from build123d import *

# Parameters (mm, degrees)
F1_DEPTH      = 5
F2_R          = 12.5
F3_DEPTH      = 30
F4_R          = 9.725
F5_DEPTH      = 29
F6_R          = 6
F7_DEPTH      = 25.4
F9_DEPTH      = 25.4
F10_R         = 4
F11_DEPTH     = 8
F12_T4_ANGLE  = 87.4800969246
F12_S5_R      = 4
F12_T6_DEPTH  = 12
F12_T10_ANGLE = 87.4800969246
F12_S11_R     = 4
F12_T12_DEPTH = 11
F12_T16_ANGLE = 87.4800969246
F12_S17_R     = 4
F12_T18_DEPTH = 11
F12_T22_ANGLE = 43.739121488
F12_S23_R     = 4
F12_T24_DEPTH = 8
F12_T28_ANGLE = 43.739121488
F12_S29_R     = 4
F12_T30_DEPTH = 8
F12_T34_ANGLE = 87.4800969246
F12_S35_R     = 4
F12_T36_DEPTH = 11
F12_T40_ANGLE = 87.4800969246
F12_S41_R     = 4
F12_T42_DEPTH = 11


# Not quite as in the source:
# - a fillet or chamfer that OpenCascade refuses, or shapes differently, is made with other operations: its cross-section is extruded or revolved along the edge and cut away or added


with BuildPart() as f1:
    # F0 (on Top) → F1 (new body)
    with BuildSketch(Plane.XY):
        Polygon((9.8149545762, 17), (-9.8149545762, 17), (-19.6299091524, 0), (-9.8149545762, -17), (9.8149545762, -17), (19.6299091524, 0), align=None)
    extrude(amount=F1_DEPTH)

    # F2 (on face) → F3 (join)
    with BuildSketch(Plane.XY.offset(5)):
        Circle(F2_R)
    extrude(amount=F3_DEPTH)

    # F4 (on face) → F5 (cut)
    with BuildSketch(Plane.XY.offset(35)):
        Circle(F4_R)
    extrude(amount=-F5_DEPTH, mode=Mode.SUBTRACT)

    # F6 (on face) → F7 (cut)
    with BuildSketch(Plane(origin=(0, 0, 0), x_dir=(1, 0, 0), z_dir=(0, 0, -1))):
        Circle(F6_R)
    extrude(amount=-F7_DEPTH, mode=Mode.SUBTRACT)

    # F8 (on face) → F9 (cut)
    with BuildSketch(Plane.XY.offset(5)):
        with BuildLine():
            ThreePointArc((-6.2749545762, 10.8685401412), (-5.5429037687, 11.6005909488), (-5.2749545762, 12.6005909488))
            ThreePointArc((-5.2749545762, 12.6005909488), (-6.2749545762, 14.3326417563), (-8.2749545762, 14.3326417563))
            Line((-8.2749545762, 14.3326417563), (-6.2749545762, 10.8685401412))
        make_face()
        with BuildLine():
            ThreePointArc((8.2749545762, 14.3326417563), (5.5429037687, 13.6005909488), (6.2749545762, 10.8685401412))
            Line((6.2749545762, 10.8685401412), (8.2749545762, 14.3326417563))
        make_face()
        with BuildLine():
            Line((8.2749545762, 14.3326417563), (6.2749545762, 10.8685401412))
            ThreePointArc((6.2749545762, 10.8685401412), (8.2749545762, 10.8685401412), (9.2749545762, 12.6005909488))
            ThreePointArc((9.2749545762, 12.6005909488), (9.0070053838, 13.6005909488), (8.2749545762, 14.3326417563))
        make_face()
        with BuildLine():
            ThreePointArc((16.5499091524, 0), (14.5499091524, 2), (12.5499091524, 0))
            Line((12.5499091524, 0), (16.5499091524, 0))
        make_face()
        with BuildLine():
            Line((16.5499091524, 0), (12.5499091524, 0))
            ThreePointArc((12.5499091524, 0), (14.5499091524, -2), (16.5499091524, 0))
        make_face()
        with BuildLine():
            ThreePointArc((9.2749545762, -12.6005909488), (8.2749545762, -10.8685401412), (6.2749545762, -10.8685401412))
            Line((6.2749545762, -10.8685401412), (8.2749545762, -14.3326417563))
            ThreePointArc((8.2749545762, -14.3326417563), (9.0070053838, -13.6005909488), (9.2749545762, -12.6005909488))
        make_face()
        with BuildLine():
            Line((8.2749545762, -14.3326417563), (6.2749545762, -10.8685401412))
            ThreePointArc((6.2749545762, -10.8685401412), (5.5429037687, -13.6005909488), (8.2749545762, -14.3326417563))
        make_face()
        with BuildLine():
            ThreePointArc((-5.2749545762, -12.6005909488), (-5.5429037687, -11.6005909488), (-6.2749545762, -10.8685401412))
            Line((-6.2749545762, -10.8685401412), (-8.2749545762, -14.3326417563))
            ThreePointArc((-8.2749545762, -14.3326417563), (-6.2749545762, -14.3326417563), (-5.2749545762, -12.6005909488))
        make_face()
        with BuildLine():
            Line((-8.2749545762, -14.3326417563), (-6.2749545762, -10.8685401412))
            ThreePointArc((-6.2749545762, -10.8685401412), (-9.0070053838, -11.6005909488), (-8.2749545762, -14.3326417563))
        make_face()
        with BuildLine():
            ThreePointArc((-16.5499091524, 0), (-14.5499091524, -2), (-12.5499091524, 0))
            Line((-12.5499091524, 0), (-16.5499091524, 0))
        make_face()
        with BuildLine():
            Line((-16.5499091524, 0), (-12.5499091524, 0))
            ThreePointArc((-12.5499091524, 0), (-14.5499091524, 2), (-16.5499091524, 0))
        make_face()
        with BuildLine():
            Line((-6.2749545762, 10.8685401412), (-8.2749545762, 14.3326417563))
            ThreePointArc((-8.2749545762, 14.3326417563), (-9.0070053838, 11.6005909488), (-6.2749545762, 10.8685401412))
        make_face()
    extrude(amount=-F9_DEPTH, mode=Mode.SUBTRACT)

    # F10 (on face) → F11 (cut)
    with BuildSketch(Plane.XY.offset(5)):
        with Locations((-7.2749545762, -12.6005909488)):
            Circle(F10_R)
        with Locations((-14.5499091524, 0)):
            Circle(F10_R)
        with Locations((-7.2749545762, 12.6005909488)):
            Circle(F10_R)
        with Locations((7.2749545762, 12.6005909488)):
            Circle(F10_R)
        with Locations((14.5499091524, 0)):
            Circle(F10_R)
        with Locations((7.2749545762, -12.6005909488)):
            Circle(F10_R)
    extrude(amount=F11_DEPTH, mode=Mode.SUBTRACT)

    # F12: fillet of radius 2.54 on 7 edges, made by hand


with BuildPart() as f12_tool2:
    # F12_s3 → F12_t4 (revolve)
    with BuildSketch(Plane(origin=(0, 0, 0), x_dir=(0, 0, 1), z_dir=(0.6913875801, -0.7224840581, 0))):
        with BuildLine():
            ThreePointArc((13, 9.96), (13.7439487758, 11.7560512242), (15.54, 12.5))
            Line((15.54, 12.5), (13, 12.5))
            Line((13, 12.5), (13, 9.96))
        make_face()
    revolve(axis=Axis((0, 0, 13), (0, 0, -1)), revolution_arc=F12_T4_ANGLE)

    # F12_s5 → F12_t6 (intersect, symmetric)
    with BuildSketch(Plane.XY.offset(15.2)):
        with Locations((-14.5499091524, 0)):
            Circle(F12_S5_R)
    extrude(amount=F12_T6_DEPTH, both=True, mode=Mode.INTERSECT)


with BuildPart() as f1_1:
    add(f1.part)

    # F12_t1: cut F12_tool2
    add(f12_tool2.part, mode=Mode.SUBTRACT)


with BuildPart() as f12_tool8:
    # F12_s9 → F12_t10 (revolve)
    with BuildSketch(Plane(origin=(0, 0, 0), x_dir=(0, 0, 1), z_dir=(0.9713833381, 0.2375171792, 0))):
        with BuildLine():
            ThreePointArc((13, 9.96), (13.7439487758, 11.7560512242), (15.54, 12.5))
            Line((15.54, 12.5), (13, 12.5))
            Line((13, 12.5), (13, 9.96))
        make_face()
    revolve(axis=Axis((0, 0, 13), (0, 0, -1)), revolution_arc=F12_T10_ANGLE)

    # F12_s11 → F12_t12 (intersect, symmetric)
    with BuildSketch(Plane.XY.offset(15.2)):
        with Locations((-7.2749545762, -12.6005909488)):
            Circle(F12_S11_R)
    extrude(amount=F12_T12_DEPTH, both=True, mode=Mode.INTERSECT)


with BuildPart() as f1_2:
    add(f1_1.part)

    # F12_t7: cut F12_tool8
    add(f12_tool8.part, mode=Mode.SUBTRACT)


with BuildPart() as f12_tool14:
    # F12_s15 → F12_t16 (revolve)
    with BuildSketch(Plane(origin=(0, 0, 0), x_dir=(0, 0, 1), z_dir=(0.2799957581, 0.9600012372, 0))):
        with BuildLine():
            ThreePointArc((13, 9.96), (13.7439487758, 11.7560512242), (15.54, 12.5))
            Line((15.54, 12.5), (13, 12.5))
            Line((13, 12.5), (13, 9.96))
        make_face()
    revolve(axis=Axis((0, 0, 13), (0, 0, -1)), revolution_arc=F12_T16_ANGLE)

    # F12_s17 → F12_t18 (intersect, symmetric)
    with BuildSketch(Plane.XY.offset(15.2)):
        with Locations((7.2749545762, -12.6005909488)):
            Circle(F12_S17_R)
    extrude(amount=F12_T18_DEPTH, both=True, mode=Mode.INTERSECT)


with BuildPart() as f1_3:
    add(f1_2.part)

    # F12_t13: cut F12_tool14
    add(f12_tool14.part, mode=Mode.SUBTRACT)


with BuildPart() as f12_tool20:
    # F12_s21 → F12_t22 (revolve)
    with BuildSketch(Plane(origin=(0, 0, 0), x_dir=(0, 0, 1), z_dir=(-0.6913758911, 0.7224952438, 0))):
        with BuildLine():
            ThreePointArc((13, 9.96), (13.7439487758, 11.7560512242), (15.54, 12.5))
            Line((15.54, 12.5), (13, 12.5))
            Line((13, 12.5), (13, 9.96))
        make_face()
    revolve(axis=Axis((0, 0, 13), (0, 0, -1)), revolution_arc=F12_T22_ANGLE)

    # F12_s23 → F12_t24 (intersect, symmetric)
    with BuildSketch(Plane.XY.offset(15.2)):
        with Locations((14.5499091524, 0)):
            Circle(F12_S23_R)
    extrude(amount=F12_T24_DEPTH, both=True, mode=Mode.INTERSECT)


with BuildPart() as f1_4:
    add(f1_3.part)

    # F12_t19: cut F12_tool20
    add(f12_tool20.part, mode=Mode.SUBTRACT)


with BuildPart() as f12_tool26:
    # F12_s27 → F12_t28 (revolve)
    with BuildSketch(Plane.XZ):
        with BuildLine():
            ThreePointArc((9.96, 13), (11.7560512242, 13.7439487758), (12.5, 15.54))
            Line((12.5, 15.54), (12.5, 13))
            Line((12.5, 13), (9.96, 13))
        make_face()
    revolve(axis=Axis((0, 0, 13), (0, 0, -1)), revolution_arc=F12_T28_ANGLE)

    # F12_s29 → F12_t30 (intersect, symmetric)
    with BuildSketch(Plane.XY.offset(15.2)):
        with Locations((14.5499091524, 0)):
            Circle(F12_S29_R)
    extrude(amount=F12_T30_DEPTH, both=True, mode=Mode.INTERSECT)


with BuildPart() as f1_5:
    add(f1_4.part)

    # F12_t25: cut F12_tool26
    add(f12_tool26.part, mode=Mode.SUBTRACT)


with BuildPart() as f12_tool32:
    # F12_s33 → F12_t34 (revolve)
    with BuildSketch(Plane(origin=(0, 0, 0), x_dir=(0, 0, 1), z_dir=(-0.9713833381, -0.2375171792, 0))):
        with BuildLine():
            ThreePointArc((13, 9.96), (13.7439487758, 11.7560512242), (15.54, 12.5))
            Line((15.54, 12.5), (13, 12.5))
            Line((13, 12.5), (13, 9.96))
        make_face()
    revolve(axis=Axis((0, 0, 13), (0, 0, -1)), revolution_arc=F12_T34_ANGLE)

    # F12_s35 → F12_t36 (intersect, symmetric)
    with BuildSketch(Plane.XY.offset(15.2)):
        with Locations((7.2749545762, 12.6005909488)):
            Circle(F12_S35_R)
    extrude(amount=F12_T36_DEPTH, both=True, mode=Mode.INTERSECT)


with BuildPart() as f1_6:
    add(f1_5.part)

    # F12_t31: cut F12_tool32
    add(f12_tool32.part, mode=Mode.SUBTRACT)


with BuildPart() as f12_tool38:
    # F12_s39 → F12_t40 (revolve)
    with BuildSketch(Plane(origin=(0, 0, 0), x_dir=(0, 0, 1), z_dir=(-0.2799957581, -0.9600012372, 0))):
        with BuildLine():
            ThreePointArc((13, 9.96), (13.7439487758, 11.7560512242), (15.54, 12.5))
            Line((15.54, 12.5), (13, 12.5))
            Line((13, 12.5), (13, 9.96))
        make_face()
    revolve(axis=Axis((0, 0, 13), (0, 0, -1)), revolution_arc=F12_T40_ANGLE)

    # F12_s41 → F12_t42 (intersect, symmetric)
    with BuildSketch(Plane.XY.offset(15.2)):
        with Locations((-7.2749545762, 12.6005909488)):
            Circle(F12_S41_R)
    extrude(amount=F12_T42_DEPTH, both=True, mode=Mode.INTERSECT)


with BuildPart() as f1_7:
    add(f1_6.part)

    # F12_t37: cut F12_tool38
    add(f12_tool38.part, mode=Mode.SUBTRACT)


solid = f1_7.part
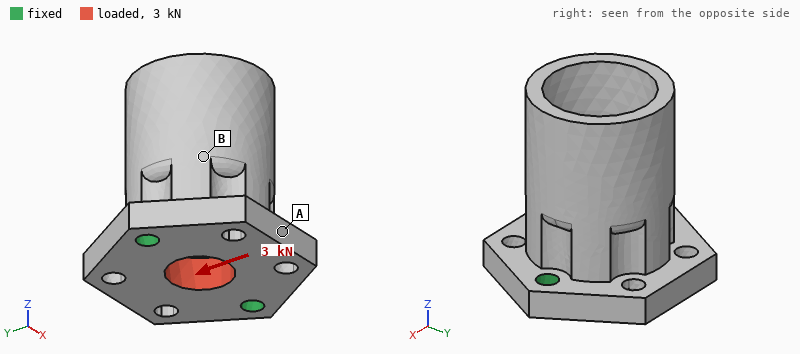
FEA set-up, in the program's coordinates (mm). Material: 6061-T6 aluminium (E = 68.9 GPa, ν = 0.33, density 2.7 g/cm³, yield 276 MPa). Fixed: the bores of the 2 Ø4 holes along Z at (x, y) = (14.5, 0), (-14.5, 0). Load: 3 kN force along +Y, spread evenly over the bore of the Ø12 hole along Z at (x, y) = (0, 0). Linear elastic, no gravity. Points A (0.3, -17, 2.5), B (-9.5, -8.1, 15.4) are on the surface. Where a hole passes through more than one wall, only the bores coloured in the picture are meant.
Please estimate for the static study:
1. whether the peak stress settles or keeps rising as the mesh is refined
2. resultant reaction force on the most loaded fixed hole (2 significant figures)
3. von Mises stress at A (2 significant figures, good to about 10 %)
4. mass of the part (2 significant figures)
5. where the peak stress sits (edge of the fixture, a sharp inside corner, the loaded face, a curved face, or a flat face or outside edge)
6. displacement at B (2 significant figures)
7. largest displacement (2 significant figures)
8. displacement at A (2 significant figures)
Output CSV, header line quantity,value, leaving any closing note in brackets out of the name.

quantity,value
whether the peak stress settles or keeps rising as the mesh is refined,keeps rising
resultant reaction force on the most loaded fixed hole,1.5 kN
von Mises stress at A,16 MPa
mass of the part,26 g
where the peak stress sits,edge of the fixture
displacement at B,6.7 µm
largest displacement,11 µm
displacement at A,6.5 µm
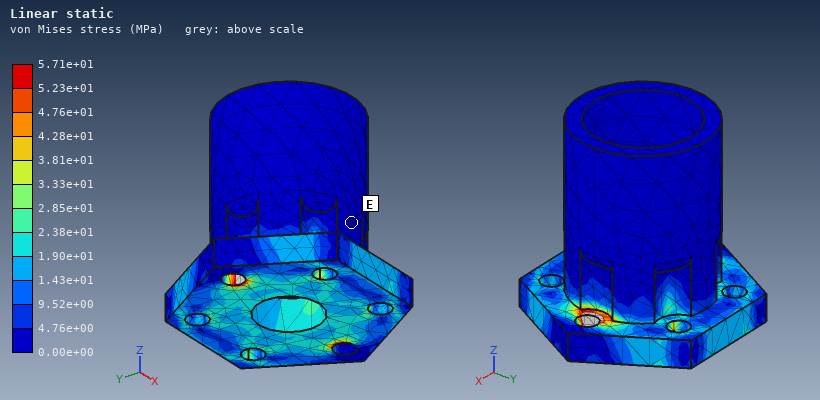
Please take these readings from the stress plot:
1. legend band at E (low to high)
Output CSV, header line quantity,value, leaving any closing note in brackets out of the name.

quantity,value
legend band at E,0.00e+00 to 4.76e+00 MPa
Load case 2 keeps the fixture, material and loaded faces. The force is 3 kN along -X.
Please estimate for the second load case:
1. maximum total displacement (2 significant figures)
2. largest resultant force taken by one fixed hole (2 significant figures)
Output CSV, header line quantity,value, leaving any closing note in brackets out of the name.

quantity,value
maximum total displacement,4.7 µm
largest resultant force taken by one fixed hole,1.5 kN
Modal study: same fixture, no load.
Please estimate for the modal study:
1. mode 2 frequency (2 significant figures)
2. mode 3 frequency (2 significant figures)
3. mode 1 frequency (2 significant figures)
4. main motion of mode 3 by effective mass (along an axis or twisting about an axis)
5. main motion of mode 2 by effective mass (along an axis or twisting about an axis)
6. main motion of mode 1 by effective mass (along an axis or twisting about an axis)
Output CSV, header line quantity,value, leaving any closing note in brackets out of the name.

quantity,value
mode 2 frequency,10 kHz
mode 3 frequency,14 kHz
mode 1 frequency,4400 Hz
main motion of mode 3 by effective mass,along Z
main motion of mode 2 by effective mass,along X
main motion of mode 1 by effective mass,along Y
